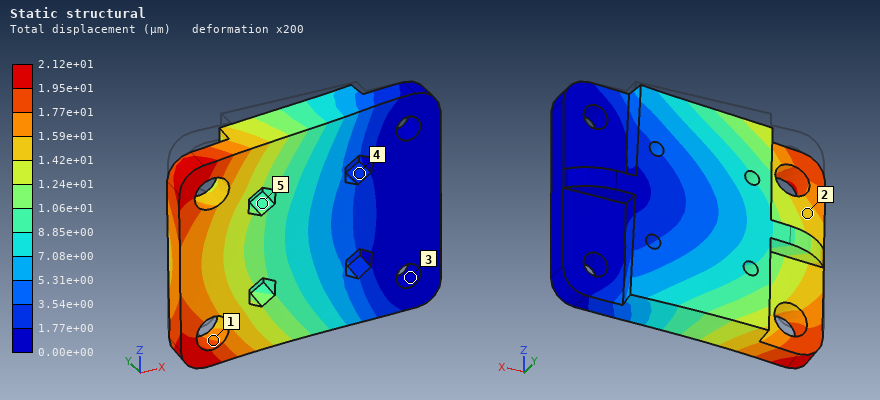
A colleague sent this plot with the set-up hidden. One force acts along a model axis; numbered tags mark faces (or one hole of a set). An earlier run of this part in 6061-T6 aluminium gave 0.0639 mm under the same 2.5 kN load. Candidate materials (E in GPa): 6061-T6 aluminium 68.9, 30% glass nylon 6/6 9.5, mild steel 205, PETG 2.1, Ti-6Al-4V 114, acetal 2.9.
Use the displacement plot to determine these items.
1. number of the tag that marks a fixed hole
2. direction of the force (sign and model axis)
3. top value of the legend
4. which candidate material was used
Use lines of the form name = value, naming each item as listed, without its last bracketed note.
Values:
number of the tag that marks a fixed hole = 3
direction of the force = -Z
top value of the legend = 2.12e+01 µm
which candidate material was used = mild steel
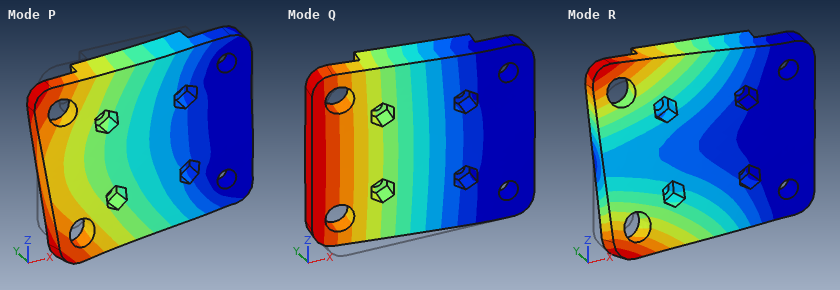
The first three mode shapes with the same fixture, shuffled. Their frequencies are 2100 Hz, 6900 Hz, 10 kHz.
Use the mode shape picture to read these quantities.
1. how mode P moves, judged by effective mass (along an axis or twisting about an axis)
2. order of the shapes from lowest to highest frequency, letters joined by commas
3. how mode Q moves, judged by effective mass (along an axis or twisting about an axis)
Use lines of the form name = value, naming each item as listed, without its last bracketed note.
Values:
how mode P moves, judged by effective mass = along Z
order of the shapes from lowest to highest frequency, letters joined by commas = Q, R, P
how mode Q moves, judged by effective mass = along Y
